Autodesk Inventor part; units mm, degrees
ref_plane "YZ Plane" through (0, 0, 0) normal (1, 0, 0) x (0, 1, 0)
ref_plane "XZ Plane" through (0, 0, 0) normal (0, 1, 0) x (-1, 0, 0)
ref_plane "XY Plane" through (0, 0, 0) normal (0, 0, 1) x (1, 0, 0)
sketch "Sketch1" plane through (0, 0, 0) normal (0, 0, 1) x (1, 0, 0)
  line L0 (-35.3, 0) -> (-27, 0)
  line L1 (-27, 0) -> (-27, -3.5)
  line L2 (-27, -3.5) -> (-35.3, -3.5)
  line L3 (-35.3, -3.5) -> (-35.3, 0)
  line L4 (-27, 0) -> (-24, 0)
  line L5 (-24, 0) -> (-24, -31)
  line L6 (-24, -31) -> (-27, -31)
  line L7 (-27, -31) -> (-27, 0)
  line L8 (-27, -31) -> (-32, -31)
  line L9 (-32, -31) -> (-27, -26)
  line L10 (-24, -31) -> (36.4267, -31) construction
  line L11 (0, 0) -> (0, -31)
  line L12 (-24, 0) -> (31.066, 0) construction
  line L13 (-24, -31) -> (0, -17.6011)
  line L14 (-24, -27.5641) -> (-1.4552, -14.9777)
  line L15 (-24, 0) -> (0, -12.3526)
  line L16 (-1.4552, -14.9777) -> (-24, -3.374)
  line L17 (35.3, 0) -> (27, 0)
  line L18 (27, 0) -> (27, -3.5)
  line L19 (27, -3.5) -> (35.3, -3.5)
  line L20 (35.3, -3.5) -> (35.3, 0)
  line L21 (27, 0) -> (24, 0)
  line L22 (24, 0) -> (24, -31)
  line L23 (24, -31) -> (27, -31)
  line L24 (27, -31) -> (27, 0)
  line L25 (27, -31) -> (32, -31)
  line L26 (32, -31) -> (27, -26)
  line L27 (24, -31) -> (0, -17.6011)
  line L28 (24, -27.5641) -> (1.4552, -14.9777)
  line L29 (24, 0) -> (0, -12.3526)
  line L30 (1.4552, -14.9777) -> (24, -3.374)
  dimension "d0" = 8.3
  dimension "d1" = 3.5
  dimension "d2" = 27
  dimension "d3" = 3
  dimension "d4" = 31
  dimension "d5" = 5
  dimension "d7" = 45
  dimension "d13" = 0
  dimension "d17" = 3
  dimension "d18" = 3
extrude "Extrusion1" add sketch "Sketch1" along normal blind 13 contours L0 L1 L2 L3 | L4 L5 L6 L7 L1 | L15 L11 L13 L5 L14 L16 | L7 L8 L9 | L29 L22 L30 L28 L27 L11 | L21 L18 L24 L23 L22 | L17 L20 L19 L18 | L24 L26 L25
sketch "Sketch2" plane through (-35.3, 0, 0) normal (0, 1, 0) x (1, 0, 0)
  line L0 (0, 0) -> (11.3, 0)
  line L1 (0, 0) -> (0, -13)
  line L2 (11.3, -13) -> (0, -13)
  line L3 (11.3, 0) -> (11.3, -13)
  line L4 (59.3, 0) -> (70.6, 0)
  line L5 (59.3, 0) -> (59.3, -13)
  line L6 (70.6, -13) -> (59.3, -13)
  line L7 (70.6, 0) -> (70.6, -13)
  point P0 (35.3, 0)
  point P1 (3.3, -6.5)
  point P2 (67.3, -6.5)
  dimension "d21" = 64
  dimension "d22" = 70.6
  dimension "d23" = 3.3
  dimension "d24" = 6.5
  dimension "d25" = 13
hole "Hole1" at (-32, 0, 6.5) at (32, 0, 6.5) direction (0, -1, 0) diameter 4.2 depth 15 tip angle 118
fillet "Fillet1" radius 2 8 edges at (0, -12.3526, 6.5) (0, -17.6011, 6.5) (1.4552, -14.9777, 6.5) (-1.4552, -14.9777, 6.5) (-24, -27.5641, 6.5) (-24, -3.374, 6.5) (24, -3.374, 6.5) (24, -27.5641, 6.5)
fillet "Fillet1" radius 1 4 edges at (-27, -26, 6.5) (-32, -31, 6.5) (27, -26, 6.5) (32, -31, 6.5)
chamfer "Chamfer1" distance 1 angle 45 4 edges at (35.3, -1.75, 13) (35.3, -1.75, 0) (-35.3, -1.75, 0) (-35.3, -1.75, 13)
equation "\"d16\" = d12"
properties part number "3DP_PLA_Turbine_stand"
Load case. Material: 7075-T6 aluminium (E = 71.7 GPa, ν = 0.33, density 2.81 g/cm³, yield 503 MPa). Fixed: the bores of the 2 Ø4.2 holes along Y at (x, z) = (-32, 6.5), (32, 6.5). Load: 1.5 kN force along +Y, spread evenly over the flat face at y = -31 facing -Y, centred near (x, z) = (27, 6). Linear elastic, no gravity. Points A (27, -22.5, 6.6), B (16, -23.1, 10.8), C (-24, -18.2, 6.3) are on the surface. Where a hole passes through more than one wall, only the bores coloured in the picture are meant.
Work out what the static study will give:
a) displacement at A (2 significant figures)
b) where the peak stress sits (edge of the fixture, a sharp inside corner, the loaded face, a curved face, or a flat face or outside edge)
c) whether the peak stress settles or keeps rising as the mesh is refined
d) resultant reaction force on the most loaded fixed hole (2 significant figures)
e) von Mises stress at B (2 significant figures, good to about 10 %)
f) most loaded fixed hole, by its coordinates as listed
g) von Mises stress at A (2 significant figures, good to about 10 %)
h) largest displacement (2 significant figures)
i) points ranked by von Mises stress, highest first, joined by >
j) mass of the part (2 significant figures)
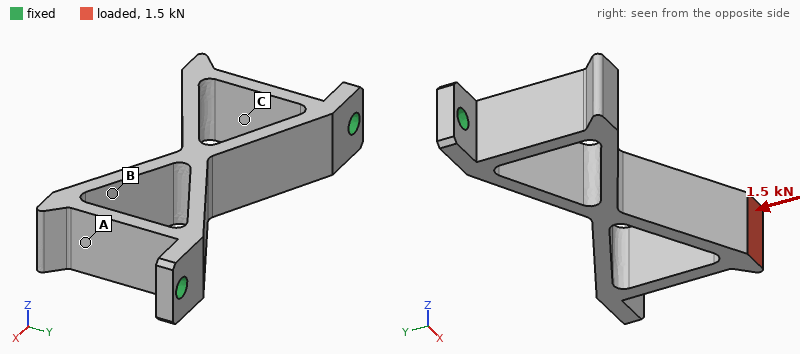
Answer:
38 µm
edge of the fixture
keeps rising
1.5 kN
28 MPa
(32, 6.5)
69 MPa
62 µm
A > B > C
22 g
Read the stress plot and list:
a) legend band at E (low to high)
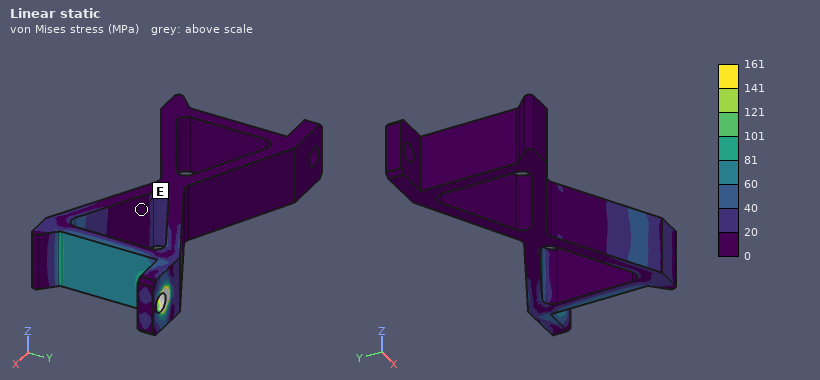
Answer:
0 to 20 MPa
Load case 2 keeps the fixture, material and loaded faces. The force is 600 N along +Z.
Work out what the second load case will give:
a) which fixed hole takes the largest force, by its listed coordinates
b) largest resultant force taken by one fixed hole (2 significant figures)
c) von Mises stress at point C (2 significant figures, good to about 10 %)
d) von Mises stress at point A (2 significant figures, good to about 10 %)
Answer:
(32, 6.5)
560 N
31 MPa
34 MPa
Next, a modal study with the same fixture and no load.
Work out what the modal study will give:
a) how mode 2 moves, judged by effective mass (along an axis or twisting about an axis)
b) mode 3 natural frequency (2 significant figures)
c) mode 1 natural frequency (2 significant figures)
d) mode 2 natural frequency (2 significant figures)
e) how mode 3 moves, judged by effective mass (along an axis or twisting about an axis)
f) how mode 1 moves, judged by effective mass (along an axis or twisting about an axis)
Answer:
twisting about Y
7900 Hz
2800 Hz
6200 Hz
along Y
along Z
